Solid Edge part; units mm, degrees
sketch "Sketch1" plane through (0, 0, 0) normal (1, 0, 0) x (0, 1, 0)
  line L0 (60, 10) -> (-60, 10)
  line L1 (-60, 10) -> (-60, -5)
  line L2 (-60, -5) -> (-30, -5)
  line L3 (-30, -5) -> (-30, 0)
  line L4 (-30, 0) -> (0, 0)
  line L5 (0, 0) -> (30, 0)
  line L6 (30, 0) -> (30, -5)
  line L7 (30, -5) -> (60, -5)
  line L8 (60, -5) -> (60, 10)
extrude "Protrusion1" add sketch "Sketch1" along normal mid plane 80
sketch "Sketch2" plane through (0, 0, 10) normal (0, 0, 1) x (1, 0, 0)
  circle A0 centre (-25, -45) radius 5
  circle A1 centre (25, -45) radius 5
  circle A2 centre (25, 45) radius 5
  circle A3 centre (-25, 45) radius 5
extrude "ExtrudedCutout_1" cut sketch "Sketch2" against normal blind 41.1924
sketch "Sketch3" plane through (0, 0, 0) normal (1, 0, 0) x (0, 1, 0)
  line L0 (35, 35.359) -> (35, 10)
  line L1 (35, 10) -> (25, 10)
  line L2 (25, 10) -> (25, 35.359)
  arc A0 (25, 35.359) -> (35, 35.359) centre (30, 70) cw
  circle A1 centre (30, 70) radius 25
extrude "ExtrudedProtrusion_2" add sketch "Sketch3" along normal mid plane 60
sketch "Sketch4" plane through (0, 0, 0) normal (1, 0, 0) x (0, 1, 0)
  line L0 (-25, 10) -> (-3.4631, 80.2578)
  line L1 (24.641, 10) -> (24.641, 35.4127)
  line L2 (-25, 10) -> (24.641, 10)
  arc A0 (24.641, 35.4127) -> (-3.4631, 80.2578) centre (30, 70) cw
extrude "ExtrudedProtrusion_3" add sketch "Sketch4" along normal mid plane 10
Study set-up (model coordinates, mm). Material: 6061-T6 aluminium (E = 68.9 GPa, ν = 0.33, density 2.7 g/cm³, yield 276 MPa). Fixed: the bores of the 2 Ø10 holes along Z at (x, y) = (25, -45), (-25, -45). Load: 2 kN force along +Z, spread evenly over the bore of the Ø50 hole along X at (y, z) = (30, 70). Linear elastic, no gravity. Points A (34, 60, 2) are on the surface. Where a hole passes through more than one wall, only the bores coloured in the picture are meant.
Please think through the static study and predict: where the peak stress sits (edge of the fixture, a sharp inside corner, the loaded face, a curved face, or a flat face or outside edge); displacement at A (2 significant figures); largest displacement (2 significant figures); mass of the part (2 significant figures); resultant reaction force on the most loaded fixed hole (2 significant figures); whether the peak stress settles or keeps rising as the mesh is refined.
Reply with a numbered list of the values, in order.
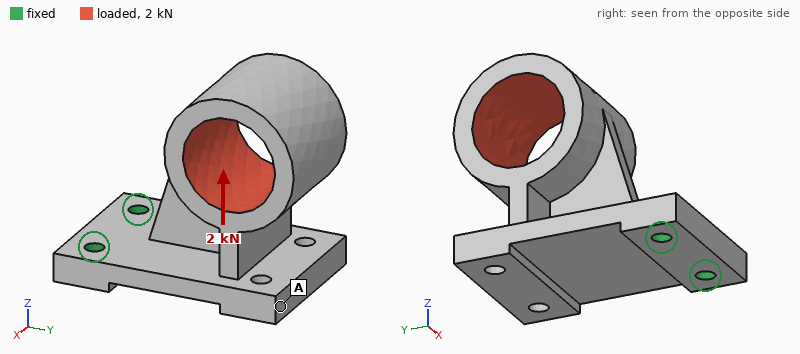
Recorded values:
1. edge of the fixture
2. 0.52 mm
3. 0.73 mm
4. 700 g
5. 1.0 kN
6. keeps rising
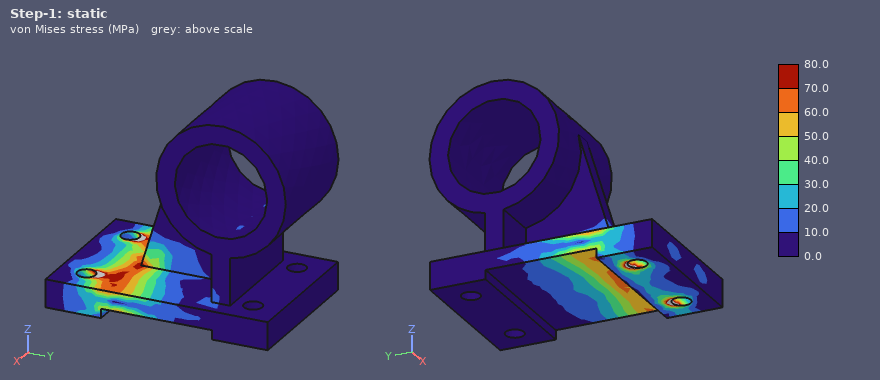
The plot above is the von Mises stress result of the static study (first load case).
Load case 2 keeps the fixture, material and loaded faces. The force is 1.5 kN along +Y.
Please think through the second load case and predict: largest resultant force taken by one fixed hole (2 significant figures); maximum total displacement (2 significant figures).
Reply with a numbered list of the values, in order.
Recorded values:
1. 830 N
2. 0.65 mm
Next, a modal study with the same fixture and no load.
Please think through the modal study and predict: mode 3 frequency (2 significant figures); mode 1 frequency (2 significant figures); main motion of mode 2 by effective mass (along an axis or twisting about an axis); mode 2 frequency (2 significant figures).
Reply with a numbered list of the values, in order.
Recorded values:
1. 2300 Hz
2. 370 Hz
3. along X
4. 590 Hz
